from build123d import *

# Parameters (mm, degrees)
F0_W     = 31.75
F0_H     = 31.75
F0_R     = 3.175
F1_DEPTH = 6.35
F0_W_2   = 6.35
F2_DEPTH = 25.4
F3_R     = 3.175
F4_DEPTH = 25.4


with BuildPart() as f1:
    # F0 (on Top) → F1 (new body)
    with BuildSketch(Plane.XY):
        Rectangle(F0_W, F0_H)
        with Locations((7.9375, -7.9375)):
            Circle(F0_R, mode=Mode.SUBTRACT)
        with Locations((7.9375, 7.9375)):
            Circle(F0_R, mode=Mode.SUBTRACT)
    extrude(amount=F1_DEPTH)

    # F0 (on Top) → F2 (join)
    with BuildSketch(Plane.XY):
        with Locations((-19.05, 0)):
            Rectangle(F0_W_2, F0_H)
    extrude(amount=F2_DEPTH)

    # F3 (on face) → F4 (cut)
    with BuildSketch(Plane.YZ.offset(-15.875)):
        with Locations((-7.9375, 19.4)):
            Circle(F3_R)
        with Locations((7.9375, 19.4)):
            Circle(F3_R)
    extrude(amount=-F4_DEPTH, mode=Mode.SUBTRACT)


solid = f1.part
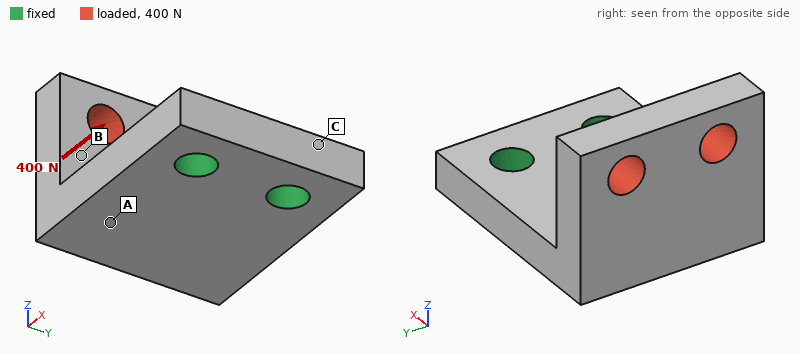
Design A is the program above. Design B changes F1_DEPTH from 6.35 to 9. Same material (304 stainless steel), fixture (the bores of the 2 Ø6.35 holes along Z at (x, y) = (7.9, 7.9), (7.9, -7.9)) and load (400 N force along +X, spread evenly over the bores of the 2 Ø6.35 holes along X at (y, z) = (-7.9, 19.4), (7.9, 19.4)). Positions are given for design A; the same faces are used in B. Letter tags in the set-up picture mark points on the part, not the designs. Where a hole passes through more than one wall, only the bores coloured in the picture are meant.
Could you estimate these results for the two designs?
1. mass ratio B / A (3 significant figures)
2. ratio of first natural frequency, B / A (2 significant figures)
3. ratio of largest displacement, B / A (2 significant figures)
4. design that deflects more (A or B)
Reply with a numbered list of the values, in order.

1. 1.23
2. 1.6
3. 0.38
4. A
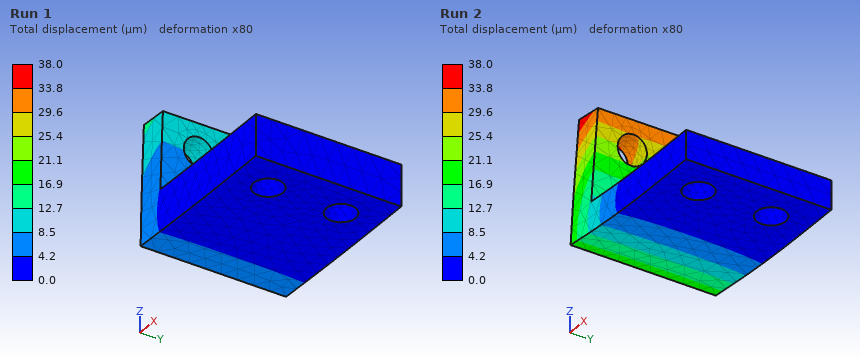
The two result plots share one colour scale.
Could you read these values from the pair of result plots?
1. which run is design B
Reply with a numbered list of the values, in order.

1. Run 1
